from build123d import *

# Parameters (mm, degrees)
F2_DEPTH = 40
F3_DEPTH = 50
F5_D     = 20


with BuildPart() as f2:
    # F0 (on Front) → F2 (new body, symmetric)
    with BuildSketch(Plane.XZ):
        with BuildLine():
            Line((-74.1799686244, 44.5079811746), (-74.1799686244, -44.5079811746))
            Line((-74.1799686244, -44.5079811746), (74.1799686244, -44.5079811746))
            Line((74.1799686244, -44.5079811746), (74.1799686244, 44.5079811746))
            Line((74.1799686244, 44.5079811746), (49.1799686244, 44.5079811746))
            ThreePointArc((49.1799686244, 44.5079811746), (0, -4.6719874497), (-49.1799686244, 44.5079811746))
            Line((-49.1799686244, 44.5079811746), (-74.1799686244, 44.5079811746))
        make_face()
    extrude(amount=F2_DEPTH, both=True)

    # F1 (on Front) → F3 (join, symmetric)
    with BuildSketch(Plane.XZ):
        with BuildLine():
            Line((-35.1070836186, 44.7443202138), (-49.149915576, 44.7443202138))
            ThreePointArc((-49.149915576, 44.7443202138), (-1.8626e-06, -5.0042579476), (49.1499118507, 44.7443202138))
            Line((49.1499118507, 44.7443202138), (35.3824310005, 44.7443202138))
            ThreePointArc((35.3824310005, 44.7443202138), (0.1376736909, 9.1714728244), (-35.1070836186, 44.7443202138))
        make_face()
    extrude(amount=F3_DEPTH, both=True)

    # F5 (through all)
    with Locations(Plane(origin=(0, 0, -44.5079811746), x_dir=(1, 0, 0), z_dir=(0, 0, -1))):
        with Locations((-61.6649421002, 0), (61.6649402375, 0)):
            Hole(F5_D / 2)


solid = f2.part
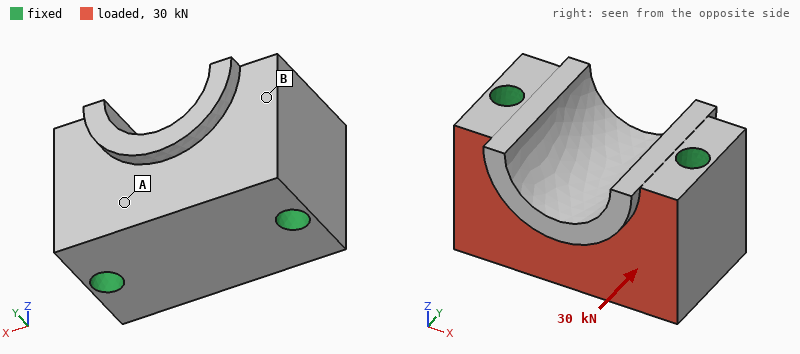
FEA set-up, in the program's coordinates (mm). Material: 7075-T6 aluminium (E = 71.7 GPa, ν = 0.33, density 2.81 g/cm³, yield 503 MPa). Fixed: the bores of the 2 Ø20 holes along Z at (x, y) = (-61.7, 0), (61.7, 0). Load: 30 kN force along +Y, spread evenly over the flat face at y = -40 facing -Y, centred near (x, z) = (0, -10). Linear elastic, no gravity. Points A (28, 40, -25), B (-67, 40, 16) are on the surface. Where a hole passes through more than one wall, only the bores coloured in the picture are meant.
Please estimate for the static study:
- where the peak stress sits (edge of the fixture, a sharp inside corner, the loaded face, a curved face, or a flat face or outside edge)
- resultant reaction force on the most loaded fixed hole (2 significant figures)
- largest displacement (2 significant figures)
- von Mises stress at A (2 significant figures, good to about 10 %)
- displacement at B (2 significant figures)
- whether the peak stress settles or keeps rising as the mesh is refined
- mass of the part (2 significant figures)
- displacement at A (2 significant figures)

edge of the fixture
15 kN
5.8 µm
2.2 MPa
1.1 µm
keeps rising
2.5 kg
2.5 µm
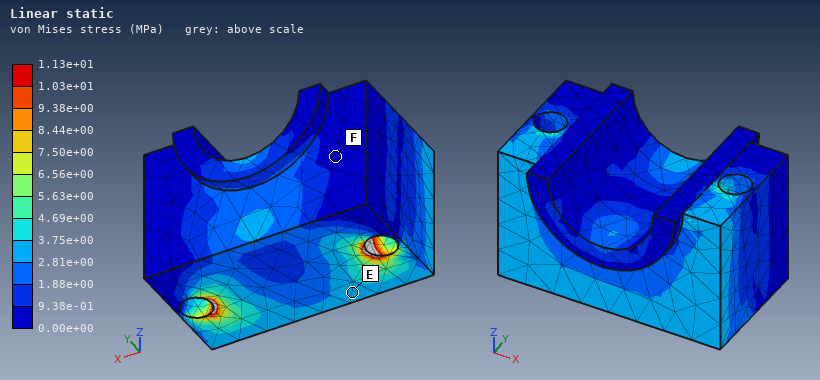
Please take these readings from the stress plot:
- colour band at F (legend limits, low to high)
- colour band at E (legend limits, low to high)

0.00e+00 to 9.38e-01 MPa
2.81e+00 to 3.75e+00 MPa
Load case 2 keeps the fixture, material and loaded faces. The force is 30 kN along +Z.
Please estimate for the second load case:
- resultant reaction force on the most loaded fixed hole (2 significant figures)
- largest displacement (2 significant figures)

15 kN
12 µm
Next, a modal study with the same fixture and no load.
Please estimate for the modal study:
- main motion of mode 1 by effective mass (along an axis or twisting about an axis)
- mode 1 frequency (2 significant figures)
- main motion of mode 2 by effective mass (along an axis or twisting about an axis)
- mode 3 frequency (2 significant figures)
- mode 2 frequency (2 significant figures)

along Y
9600 Hz
along Z
12 kHz
11 kHz
